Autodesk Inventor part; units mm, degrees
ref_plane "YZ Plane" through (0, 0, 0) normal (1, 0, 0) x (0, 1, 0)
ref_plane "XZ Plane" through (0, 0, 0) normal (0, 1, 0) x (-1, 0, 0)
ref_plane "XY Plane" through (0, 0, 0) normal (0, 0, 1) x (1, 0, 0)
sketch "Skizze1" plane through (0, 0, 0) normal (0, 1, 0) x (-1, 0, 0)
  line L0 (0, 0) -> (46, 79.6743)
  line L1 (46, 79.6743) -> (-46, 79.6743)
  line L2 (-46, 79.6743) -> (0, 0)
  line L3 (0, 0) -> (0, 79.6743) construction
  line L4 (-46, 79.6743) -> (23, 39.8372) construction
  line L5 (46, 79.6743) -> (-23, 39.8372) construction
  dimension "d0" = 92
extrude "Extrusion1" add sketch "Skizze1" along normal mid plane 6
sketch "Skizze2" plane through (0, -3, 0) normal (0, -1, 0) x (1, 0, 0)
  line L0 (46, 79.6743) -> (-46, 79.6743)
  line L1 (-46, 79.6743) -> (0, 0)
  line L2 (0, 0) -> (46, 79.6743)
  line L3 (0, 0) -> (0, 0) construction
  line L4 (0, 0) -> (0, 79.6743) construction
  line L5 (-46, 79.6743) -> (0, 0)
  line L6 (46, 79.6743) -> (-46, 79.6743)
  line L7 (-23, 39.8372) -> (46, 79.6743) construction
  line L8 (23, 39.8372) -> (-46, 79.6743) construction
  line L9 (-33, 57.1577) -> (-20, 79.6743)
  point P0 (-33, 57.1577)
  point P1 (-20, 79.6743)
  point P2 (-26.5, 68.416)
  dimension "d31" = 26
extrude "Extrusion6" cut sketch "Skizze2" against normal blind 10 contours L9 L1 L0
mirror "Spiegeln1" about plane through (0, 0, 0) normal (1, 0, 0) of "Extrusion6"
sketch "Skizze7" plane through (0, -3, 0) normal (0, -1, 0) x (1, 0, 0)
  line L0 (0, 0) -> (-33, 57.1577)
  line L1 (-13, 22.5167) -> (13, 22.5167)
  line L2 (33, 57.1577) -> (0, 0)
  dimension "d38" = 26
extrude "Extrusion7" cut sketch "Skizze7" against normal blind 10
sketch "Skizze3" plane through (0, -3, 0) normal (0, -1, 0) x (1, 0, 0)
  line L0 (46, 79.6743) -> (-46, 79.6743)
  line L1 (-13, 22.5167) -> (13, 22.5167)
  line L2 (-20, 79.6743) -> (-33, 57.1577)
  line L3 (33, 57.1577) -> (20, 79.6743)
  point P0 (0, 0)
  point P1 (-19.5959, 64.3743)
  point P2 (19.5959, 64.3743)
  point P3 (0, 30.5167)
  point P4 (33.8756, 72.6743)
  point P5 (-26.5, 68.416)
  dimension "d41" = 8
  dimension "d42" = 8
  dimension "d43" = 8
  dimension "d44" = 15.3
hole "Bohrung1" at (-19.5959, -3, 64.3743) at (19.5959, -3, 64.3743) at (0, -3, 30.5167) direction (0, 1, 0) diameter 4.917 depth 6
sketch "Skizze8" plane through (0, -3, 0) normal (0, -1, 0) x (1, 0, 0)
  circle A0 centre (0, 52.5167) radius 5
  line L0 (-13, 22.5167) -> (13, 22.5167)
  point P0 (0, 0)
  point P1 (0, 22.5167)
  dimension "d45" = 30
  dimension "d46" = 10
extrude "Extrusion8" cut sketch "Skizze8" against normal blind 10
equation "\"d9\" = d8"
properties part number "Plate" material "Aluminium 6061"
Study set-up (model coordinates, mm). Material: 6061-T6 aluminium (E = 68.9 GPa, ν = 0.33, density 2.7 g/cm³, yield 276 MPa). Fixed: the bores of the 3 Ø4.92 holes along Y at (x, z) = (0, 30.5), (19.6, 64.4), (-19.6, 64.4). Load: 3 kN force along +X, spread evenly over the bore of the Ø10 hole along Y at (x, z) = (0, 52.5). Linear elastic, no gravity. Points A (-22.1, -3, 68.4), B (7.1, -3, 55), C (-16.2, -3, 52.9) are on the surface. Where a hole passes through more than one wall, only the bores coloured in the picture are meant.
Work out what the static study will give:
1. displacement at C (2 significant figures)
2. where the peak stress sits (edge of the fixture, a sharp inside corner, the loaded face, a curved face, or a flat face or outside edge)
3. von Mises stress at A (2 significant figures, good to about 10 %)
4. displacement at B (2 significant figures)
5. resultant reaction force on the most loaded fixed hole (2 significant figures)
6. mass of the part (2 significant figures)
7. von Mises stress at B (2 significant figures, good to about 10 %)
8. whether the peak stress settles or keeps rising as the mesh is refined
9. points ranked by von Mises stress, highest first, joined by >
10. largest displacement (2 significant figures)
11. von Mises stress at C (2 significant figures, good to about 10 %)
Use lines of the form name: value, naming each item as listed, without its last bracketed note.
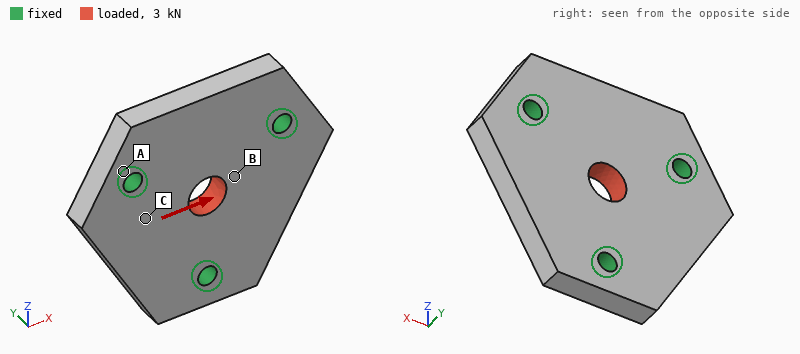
displacement at C: 2.8 µm
where the peak stress sits: edge of the fixture
von Mises stress at A: 3.7 MPa
displacement at B: 3.6 µm
resultant reaction force on the most loaded fixed hole: 1.0 kN
mass of the part: 43 g
von Mises stress at B: 16 MPa
whether the peak stress settles or keeps rising as the mesh is refined: keeps rising
points ranked by von Mises stress, highest first, joined by >: B > C > A
largest displacement: 5.3 µm
von Mises stress at C: 8.7 MPa
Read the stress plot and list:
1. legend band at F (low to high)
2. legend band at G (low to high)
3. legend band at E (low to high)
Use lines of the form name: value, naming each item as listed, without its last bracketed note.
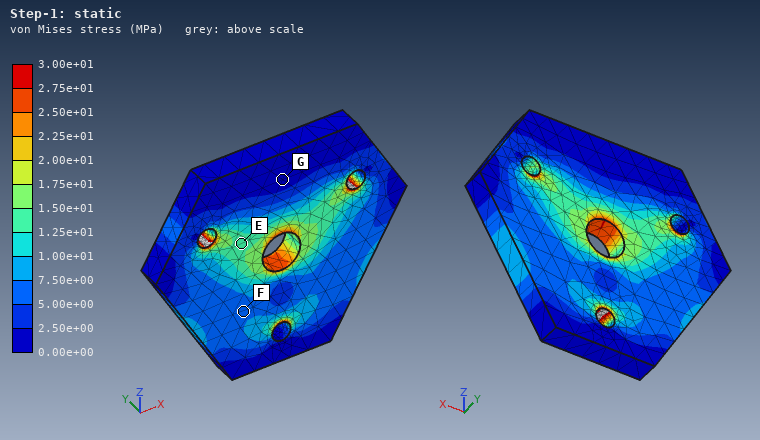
legend band at F: 5.00e+00 to 7.50e+00 MPa
legend band at G: 0.00e+00 to 2.50e+00 MPa
legend band at E: 1.25e+01 to 1.50e+01 MPa
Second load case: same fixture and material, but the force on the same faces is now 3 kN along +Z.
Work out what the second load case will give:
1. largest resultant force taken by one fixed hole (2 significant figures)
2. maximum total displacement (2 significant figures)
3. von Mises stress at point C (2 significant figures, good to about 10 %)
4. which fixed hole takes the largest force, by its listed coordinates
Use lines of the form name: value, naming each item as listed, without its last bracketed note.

largest resultant force taken by one fixed hole: 1.1 kN
maximum total displacement: 5.3 µm
von Mises stress at point C: 5.1 MPa
which fixed hole takes the largest force, by its listed coordinates: (0, 30.5)
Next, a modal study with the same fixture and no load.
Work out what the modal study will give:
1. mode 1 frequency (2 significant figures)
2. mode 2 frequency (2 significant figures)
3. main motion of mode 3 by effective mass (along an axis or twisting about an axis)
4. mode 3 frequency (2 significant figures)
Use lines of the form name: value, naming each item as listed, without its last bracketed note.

mode 1 frequency: 13 kHz
mode 2 frequency: 13 kHz
main motion of mode 3 by effective mass: along Y
mode 3 frequency: 15 kHz
